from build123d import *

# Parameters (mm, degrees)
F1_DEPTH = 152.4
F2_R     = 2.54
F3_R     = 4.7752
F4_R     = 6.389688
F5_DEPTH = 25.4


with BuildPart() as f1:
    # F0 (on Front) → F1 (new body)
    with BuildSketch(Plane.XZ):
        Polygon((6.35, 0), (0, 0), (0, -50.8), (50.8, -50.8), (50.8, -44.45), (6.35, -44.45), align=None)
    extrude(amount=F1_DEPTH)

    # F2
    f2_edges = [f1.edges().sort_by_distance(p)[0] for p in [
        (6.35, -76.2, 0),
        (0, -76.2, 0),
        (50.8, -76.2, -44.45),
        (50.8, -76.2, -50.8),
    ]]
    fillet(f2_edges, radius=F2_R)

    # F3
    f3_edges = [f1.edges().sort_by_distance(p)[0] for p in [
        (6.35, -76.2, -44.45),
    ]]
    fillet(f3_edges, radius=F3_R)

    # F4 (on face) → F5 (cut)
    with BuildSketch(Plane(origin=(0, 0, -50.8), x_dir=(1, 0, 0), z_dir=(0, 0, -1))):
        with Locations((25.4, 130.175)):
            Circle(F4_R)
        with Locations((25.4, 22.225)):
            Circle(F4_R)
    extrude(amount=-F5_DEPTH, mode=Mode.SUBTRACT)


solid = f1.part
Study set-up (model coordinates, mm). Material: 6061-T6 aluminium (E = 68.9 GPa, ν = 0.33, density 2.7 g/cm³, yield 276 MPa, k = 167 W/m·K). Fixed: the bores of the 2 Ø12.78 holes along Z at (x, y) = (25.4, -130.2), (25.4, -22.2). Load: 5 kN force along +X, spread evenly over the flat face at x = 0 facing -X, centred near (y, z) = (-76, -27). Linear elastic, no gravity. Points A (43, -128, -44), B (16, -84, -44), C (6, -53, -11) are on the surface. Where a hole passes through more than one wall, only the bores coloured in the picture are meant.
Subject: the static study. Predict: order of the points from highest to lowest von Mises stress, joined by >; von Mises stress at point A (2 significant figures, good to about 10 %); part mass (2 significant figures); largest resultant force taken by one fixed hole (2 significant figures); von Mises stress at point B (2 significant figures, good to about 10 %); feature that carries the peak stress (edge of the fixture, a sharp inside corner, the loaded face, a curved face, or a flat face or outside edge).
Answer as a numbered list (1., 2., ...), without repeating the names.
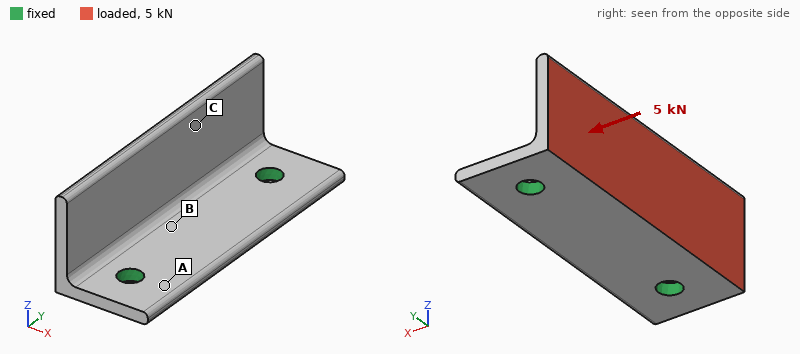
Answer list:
1. B > A > C
2. 34 MPa
3. 240 g
4. 2.5 kN
5. 58 MPa
6. a flat face or outside edge
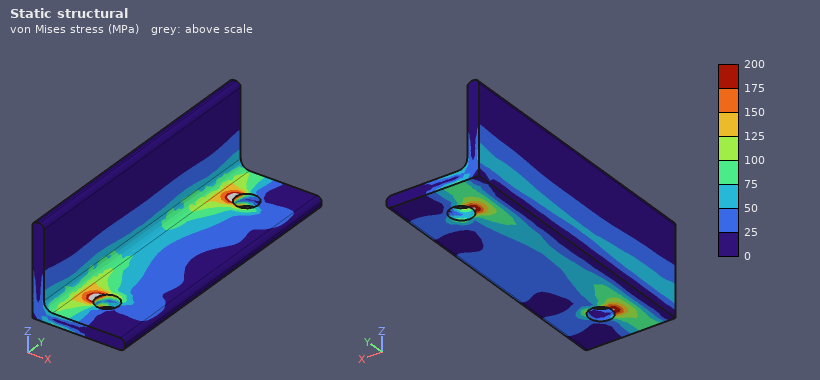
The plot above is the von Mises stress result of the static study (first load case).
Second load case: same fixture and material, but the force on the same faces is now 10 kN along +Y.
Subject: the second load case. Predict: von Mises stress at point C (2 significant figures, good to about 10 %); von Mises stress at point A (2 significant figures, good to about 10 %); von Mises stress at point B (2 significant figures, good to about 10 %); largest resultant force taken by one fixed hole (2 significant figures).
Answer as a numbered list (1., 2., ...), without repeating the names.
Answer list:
1. 11 MPa
2. 9.0 MPa
3. 24 MPa
4. 5.7 kN
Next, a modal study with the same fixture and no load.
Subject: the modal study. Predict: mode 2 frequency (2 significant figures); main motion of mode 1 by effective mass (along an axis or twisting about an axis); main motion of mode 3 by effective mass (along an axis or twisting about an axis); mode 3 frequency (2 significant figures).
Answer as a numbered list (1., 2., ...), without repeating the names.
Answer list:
1. 2100 Hz
2. along X
3. along Z
4. 3500 Hz
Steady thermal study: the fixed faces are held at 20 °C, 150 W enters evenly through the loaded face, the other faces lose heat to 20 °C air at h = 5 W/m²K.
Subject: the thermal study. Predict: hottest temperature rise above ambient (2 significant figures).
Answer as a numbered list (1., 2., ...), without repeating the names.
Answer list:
1. 47 K
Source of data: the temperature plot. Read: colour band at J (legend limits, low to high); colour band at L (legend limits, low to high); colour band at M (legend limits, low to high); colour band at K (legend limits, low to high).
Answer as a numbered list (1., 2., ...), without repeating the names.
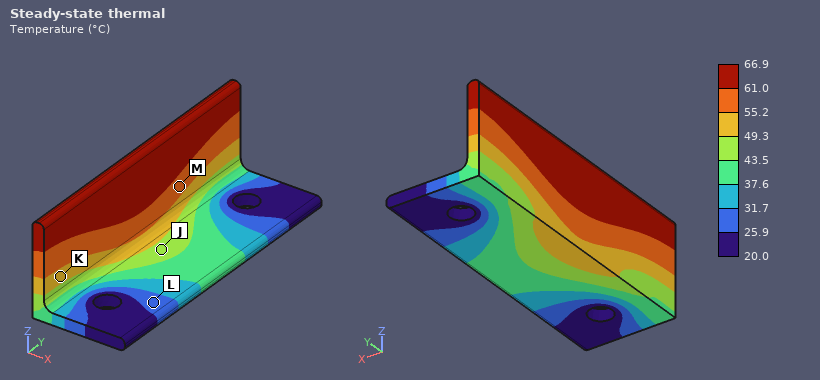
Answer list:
1. 43.5 to 49.3 °C
2. 25.9 to 31.7 °C
3. 55.2 to 61.0 °C
4. 49.3 to 55.2 °C
